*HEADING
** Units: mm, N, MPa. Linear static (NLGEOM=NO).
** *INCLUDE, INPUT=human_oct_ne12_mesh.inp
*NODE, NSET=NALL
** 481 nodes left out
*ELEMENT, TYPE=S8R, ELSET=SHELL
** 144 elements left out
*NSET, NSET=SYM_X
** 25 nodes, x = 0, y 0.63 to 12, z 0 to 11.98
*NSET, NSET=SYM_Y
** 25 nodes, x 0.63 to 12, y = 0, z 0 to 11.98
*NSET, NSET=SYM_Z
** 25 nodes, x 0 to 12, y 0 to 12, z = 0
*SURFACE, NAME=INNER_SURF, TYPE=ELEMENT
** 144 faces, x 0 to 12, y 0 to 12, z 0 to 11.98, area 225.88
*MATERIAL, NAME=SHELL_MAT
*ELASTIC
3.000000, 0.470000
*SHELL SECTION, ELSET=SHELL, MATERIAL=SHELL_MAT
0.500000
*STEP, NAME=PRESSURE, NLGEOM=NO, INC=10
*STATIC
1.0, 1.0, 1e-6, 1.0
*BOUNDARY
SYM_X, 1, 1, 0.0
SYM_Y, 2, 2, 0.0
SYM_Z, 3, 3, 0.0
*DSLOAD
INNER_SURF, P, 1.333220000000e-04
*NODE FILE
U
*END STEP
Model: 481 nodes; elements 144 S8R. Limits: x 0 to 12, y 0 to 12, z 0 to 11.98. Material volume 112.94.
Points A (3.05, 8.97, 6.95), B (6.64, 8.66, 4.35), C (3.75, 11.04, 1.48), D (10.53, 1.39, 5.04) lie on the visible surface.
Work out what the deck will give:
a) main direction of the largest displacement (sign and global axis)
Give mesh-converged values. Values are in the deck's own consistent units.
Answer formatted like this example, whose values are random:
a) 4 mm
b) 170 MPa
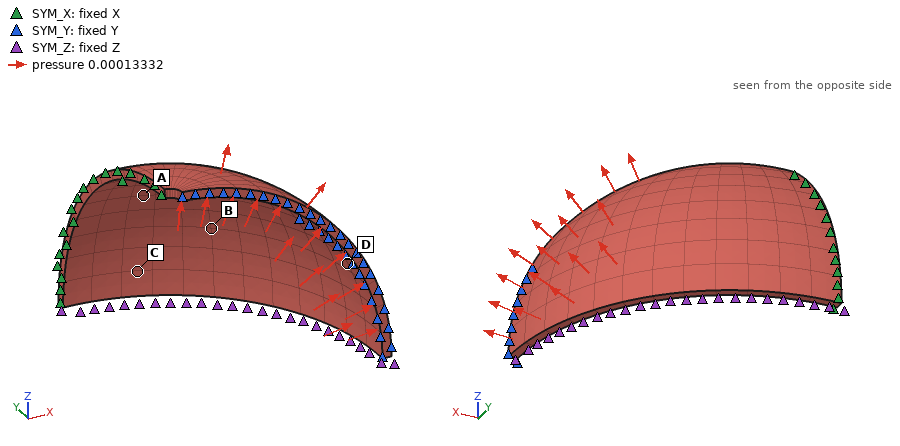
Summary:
a) +X
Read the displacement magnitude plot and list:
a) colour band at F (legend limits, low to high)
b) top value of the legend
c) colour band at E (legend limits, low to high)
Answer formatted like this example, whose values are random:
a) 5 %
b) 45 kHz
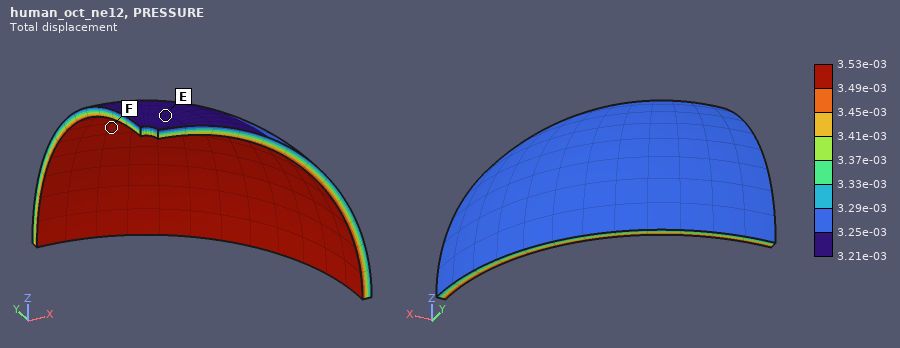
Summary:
a) 3.49e-03 to 3.53e-03
b) 3.53e-03
c) 3.21e-03 to 3.25e-03
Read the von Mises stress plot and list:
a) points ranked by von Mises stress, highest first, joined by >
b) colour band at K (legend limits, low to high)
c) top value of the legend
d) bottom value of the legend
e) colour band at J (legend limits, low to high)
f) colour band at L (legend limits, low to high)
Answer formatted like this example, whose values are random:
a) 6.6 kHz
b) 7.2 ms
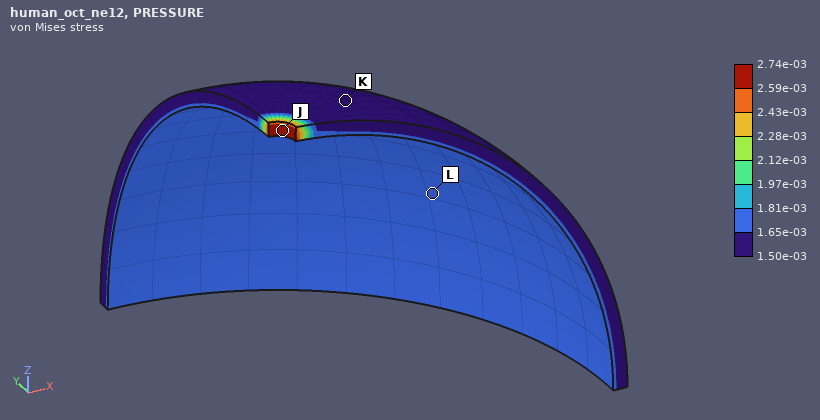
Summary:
a) J > L > K
b) 1.50e-03 to 1.65e-03
c) 2.74e-03
d) 1.50e-03
e) 2.59e-03 to 2.74e-03
f) 1.65e-03 to 1.81e-03
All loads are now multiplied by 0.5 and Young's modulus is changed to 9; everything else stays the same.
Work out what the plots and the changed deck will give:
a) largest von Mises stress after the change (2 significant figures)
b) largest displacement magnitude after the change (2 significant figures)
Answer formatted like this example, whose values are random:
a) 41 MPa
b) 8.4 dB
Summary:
a) 0.0014
b) 5.9e-04
